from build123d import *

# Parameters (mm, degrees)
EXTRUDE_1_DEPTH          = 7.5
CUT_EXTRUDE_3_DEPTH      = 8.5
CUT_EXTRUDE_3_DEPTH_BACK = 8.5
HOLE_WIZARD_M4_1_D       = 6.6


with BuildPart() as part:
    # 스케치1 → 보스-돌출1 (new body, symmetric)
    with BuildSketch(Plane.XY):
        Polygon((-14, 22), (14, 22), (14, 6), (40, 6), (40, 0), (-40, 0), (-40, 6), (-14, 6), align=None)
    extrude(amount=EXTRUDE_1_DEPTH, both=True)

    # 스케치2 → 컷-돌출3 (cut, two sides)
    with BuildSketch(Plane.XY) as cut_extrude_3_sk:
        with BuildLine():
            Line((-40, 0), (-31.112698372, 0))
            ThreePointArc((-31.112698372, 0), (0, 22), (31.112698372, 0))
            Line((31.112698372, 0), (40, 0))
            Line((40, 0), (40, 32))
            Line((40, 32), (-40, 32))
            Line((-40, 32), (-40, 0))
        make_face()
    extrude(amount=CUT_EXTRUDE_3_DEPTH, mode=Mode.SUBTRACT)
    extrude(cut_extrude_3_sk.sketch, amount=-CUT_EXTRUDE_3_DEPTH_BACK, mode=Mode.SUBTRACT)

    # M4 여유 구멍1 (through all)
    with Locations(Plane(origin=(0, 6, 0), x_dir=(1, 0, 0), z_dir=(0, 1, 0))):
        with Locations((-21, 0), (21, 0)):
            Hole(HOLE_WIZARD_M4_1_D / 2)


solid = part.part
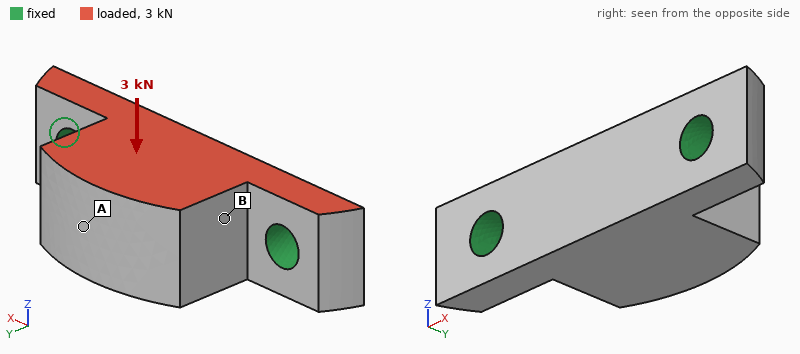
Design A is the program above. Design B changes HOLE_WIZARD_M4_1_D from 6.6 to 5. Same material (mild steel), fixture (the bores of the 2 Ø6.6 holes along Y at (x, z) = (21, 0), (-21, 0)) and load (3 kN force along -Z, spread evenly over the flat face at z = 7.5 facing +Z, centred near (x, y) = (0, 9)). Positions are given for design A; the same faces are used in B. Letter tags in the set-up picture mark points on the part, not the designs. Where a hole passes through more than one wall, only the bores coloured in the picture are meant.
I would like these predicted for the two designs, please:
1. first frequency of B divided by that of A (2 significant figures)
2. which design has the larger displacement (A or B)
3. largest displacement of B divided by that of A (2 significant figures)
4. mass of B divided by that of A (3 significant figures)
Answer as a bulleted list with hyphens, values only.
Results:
- 0.91
- B
- 1.2
- 1.02
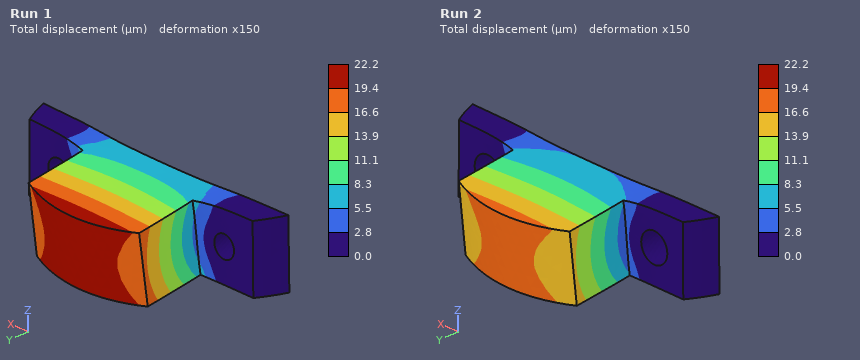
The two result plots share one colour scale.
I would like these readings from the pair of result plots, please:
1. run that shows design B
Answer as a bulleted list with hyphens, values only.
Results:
- Run 1
